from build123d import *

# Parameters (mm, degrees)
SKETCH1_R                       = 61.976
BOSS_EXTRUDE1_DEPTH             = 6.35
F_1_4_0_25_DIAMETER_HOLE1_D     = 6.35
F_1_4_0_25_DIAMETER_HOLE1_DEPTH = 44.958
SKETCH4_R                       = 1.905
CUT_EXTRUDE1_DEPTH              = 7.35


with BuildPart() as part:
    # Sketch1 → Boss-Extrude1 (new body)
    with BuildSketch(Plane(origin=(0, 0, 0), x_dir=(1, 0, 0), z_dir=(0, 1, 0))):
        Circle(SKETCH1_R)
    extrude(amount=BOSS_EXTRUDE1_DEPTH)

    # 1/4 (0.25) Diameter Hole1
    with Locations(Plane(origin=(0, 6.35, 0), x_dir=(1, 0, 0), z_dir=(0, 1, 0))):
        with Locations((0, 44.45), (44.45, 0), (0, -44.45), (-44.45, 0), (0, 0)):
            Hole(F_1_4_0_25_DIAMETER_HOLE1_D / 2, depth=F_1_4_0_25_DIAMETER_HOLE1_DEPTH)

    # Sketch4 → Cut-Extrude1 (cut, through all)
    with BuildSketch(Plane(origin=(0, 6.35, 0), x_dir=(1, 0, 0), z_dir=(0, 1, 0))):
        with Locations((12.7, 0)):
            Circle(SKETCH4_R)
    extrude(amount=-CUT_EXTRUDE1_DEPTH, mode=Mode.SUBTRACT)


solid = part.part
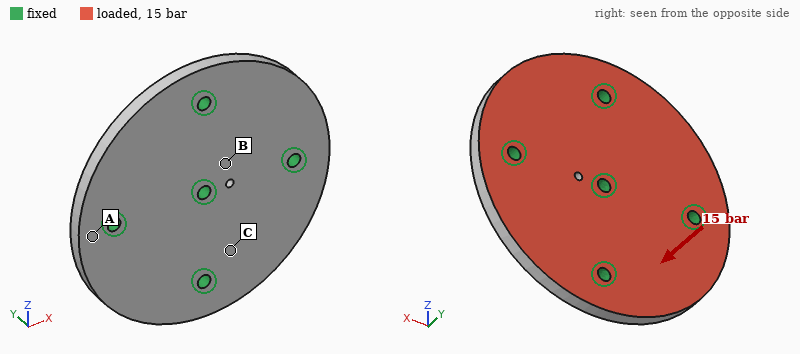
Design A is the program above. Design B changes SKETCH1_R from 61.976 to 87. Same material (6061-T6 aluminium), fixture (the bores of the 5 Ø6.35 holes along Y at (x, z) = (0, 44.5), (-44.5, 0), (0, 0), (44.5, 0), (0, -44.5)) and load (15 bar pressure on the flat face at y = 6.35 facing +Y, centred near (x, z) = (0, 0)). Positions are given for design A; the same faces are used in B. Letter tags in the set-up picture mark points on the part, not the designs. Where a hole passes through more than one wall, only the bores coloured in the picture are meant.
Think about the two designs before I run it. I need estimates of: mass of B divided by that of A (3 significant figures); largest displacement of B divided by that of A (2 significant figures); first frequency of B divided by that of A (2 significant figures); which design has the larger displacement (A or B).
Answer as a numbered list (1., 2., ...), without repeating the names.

1. 1.98
2. 6.1
3. 0.38
4. B
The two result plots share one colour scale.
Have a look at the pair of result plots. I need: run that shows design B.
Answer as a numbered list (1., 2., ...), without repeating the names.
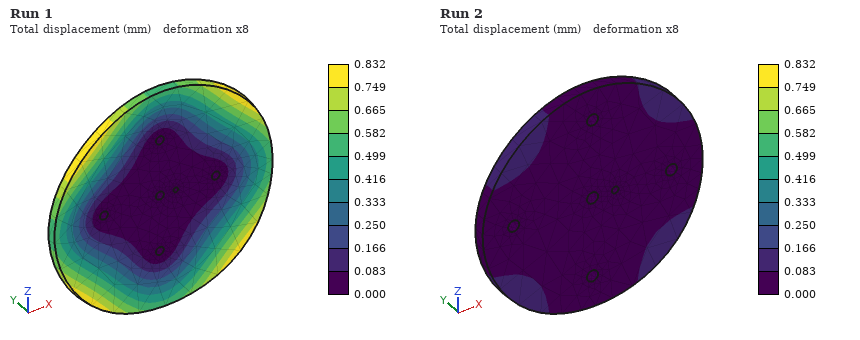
1. Run 1
